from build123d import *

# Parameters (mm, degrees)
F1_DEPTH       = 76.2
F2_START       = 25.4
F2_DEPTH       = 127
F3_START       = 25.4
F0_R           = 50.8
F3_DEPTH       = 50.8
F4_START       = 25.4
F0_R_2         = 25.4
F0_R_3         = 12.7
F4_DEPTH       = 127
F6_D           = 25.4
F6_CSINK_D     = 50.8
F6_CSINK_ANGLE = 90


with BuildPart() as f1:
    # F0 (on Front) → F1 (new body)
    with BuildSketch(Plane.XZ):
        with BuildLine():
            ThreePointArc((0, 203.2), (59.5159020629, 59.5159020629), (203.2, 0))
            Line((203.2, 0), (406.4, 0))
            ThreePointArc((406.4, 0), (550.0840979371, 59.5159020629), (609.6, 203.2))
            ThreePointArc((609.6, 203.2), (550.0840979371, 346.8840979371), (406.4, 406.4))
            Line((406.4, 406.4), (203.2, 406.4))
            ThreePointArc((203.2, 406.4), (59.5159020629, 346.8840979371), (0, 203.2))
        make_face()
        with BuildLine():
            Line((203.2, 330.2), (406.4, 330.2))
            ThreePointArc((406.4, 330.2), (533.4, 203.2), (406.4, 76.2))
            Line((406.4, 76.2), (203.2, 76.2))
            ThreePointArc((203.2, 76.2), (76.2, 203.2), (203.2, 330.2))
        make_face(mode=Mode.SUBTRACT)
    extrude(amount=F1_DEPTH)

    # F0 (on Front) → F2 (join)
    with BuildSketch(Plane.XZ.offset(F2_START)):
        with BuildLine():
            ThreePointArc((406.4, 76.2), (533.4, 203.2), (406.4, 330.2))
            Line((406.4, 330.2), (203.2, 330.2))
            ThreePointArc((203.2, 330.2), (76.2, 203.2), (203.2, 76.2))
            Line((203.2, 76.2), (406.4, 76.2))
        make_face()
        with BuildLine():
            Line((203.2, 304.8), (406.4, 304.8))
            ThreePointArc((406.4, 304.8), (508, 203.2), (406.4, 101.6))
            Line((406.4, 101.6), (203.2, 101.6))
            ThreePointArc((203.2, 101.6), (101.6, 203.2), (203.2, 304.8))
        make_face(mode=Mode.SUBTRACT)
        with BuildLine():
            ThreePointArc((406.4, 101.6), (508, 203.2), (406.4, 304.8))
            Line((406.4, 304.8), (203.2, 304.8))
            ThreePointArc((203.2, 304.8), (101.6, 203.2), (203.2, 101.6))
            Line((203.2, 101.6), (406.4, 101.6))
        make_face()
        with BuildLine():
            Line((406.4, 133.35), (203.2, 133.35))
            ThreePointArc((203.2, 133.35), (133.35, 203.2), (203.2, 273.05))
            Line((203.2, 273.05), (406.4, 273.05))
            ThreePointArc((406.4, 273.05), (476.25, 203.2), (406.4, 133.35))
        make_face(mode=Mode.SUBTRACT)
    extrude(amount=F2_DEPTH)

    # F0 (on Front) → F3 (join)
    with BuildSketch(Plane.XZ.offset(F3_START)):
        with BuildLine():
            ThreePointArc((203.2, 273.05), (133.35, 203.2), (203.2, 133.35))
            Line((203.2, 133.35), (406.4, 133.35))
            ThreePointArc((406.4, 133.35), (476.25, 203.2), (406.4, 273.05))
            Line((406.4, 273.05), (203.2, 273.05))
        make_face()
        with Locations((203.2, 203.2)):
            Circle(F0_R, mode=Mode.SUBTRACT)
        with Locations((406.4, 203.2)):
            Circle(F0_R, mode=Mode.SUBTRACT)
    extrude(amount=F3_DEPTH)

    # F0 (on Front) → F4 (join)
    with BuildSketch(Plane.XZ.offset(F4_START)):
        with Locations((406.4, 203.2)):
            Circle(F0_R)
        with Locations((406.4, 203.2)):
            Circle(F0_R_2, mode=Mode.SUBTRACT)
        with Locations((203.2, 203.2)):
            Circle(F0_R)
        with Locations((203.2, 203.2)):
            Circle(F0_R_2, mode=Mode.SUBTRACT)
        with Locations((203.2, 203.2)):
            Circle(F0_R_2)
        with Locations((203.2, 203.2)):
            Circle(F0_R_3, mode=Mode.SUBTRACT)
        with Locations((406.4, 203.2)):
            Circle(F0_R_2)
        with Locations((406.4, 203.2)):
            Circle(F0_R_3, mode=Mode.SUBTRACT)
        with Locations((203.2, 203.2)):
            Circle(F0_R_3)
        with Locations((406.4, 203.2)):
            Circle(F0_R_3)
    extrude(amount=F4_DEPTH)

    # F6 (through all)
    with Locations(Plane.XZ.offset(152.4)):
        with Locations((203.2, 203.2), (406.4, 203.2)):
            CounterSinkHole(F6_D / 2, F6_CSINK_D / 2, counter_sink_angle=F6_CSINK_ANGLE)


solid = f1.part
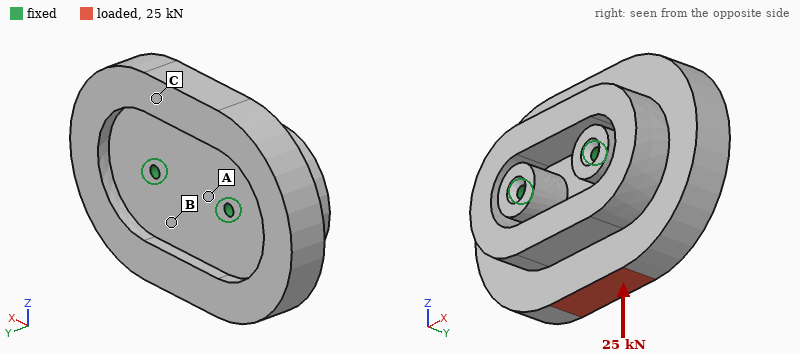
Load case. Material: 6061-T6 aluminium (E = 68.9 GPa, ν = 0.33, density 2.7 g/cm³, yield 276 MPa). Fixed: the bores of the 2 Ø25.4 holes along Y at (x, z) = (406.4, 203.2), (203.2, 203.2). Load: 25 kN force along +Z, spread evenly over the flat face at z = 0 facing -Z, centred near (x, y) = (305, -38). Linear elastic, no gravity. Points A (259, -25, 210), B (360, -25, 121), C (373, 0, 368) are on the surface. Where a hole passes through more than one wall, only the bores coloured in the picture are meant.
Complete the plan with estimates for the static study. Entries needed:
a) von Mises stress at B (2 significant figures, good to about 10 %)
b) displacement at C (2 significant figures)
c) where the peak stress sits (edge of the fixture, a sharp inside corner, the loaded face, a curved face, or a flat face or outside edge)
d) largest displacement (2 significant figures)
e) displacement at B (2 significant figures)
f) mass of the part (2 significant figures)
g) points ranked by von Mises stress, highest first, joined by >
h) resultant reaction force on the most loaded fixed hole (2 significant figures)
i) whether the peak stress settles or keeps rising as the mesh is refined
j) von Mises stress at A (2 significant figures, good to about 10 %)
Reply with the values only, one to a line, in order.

2.9 MPa
4.7 µm
edge of the fixture
20 µm
5.7 µm
52 kg
B > A > C
13 kN
keeps rising
1.0 MPa
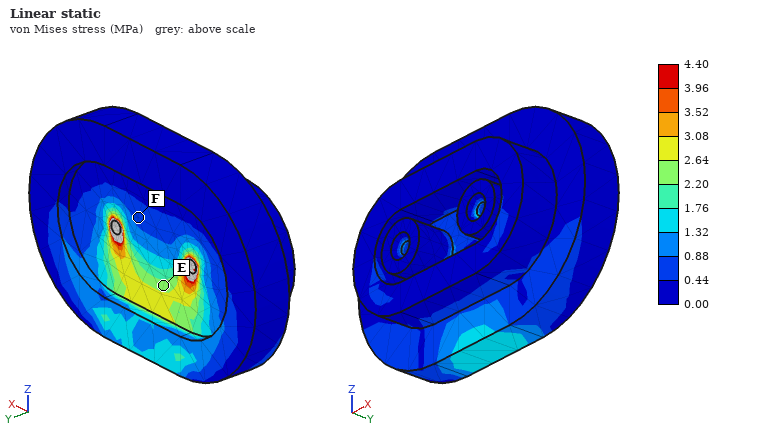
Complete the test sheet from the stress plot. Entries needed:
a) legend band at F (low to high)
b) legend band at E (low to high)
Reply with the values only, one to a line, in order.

0.44 to 0.88 MPa
2.20 to 2.64 MPa
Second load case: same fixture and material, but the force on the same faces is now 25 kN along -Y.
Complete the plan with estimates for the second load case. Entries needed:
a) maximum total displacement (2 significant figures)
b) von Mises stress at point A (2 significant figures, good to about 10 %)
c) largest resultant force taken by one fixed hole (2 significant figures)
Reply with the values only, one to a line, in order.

0.14 mm
3.4 MPa
13 kN
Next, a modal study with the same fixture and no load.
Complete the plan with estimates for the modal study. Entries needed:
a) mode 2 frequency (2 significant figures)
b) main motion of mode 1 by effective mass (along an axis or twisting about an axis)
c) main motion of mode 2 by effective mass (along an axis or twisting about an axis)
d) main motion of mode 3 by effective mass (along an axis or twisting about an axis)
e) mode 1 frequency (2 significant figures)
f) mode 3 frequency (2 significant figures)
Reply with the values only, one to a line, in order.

1200 Hz
twisting about X
twisting about Z
twisting about Y
780 Hz
1300 Hz
